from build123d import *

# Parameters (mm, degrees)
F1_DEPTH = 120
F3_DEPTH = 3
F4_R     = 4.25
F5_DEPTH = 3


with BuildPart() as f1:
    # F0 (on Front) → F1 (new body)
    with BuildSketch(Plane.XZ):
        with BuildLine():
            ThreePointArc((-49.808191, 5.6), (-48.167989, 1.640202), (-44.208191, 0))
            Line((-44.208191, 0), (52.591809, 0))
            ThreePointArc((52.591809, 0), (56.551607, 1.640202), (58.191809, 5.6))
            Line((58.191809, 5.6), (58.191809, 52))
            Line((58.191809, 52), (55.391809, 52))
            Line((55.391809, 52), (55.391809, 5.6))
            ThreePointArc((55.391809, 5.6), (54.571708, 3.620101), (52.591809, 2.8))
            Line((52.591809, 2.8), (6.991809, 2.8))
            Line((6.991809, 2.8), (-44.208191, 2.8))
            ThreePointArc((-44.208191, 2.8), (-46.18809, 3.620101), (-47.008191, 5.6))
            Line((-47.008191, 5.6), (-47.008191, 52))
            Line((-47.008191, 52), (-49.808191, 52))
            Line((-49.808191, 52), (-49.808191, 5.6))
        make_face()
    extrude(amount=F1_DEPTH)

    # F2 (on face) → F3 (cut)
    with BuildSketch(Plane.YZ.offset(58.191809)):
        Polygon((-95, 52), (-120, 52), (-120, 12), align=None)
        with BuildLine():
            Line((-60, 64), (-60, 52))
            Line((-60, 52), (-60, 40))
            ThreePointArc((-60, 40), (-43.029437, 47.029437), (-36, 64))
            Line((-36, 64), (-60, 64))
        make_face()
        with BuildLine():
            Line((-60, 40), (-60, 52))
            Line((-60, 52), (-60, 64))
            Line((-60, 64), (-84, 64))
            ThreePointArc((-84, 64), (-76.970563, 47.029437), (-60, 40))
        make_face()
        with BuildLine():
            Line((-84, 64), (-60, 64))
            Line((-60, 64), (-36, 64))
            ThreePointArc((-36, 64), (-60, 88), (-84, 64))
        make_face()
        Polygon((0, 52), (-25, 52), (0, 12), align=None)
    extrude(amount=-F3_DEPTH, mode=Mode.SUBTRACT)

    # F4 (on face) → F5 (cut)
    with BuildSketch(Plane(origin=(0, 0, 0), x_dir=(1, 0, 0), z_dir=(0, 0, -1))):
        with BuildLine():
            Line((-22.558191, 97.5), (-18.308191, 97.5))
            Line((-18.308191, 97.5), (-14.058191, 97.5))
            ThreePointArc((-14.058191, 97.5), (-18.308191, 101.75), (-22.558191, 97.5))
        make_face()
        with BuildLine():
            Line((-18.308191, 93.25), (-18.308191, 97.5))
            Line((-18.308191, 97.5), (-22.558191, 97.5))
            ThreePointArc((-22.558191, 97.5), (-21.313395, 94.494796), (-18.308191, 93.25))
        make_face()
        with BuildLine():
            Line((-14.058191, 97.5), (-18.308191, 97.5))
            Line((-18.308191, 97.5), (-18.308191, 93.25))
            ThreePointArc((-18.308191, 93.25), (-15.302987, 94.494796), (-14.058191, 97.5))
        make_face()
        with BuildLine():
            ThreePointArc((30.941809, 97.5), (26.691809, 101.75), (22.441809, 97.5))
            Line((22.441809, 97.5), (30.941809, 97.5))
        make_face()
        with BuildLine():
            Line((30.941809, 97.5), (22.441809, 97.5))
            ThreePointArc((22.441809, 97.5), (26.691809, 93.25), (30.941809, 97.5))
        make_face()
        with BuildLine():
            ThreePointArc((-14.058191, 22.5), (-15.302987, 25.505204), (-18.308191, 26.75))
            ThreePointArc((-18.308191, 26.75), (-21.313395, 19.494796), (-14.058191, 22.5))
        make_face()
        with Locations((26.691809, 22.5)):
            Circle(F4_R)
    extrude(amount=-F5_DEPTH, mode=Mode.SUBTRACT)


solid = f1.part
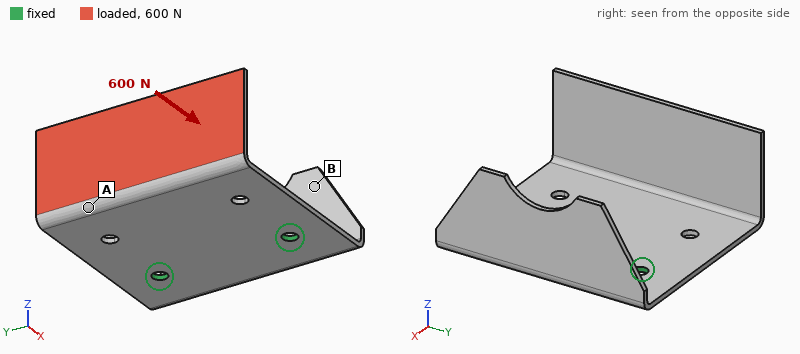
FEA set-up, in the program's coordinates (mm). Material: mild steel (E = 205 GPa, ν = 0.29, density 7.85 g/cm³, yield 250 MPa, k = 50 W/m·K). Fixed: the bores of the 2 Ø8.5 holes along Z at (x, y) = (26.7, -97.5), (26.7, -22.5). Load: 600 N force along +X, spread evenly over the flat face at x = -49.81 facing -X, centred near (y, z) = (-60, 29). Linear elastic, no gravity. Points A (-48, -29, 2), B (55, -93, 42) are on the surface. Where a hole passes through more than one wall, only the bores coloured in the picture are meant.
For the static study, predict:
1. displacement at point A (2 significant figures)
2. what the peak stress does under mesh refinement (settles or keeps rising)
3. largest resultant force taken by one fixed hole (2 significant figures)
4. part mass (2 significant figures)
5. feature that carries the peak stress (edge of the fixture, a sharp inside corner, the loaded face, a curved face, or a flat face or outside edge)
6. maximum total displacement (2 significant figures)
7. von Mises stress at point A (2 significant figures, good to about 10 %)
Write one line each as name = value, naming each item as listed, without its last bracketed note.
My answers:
displacement at point A = 1.0 mm
what the peak stress does under mesh refinement = keeps rising
largest resultant force taken by one fixed hole = 300 N
part mass = 500 g
feature that carries the peak stress = edge of the fixture
maximum total displacement = 1.9 mm
von Mises stress at point A = 76 MPa
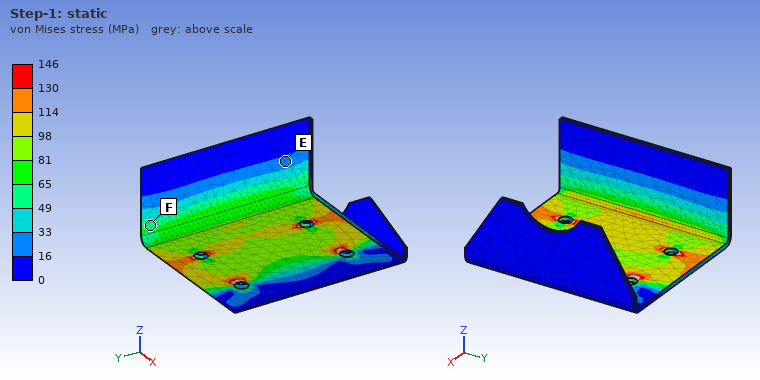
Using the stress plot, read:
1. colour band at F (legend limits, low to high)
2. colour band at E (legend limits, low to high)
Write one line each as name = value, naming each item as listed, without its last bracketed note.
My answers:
colour band at F = 49 to 65 MPa
colour band at E = 16 to 33 MPa
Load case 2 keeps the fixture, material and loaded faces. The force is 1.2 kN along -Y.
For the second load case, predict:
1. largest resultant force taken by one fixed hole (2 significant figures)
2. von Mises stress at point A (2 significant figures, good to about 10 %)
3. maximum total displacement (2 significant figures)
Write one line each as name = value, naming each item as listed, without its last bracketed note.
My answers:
largest resultant force taken by one fixed hole = 1.4 kN
von Mises stress at point A = 81 MPa
maximum total displacement = 1.4 mm
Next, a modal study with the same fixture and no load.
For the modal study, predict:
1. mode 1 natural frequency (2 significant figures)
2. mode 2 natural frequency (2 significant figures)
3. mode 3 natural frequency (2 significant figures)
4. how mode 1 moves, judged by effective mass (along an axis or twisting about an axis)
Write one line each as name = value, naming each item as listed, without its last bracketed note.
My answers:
mode 1 natural frequency = 190 Hz
mode 2 natural frequency = 370 Hz
mode 3 natural frequency = 590 Hz
how mode 1 moves, judged by effective mass = along Z
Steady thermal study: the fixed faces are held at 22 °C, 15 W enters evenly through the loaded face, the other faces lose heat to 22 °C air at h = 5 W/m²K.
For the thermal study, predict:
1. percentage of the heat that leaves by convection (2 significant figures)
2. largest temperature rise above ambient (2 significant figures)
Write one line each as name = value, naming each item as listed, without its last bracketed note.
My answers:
percentage of the heat that leaves by convection = 35 %
largest temperature rise above ambient = 74 K
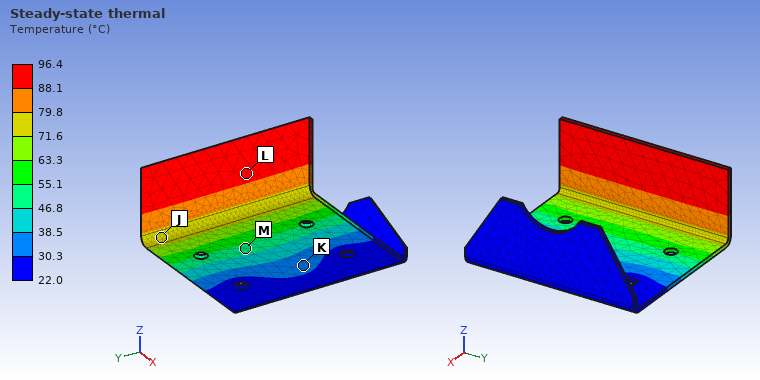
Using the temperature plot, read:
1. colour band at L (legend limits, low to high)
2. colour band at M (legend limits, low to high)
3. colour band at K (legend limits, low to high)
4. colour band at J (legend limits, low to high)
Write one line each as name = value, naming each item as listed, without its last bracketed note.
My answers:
colour band at L = 88.1 to 96.4 °C
colour band at M = 46.8 to 55.1 °C
colour band at K = 30.3 to 38.5 °C
colour band at J = 71.6 to 79.8 °C
